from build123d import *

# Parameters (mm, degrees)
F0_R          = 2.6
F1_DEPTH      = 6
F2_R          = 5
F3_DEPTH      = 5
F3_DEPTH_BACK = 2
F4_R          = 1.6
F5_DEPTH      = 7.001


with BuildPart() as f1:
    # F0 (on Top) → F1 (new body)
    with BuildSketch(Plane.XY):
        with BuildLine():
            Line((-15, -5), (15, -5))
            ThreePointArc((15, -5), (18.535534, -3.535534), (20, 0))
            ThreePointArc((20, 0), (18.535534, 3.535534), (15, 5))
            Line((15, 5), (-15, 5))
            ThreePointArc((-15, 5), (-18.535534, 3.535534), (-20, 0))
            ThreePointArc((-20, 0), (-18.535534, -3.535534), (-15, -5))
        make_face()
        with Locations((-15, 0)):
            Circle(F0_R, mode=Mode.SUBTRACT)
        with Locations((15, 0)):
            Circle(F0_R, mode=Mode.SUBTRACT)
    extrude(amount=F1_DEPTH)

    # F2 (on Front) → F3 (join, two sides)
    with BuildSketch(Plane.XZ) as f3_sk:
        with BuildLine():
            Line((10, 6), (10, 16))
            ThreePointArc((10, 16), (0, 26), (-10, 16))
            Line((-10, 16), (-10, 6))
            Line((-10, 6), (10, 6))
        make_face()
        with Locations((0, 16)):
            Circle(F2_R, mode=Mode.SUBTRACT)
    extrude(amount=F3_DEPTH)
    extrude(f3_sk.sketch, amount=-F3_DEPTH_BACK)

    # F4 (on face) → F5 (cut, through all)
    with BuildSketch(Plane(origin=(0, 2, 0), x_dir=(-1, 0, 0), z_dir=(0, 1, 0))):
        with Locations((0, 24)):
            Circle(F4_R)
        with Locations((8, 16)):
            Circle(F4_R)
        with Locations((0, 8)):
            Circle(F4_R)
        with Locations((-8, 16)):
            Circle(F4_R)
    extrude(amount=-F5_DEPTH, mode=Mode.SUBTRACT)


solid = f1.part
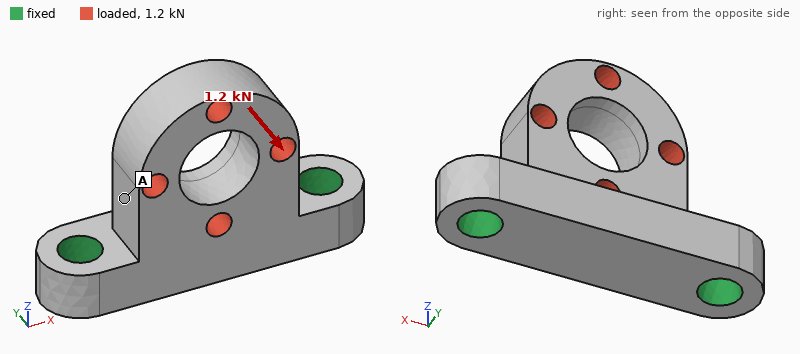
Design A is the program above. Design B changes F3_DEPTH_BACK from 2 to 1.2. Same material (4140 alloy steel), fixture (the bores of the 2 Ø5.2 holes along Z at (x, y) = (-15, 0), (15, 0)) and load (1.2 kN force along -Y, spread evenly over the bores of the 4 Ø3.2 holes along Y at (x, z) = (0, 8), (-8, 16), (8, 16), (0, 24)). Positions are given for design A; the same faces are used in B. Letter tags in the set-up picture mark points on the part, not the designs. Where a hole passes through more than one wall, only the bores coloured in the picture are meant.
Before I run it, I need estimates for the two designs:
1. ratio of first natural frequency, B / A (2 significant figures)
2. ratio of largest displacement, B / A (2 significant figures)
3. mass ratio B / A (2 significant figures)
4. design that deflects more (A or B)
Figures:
0.97
1.2
0.95
B
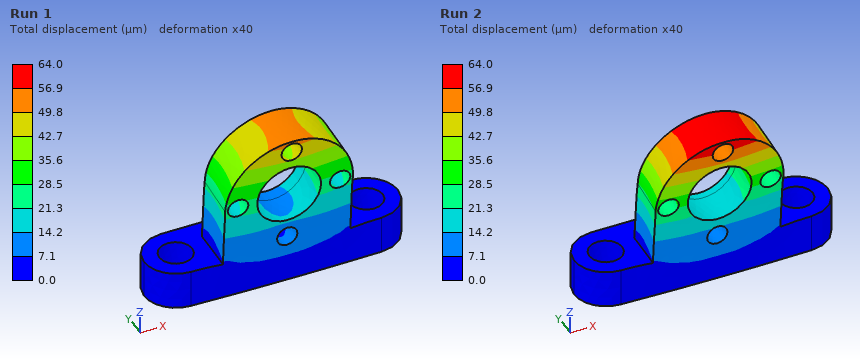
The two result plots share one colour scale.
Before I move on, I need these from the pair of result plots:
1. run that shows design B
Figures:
Run 2
